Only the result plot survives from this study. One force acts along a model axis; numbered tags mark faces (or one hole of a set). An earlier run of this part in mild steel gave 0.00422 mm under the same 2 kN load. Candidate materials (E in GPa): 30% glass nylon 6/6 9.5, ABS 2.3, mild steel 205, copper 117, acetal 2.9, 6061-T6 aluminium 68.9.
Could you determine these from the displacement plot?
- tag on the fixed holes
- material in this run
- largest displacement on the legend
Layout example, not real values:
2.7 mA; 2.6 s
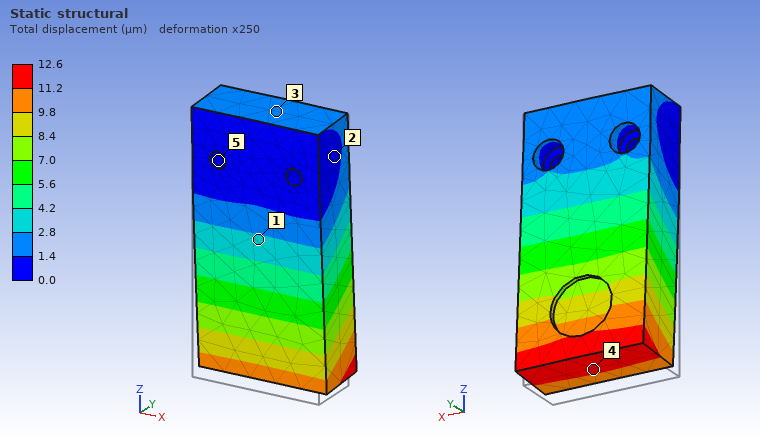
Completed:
5; 6061-T6 aluminium; 12.6 µm
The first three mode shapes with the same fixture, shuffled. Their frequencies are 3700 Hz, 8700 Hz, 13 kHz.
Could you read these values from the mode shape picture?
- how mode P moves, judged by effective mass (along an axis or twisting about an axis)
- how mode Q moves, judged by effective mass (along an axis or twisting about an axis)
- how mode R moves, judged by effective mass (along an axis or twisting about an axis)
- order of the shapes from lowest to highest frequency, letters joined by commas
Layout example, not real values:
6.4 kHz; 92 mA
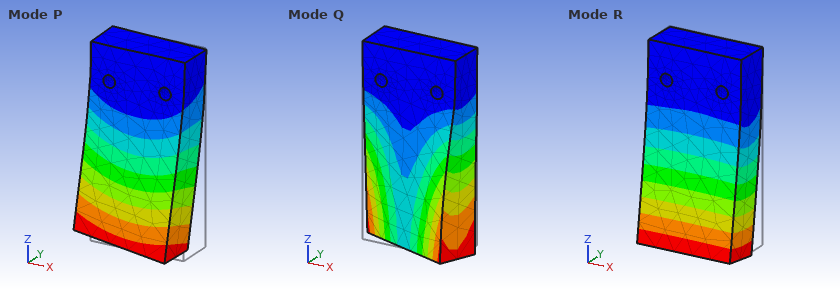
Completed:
along X; twisting about Z; along Y; R, P, Q
